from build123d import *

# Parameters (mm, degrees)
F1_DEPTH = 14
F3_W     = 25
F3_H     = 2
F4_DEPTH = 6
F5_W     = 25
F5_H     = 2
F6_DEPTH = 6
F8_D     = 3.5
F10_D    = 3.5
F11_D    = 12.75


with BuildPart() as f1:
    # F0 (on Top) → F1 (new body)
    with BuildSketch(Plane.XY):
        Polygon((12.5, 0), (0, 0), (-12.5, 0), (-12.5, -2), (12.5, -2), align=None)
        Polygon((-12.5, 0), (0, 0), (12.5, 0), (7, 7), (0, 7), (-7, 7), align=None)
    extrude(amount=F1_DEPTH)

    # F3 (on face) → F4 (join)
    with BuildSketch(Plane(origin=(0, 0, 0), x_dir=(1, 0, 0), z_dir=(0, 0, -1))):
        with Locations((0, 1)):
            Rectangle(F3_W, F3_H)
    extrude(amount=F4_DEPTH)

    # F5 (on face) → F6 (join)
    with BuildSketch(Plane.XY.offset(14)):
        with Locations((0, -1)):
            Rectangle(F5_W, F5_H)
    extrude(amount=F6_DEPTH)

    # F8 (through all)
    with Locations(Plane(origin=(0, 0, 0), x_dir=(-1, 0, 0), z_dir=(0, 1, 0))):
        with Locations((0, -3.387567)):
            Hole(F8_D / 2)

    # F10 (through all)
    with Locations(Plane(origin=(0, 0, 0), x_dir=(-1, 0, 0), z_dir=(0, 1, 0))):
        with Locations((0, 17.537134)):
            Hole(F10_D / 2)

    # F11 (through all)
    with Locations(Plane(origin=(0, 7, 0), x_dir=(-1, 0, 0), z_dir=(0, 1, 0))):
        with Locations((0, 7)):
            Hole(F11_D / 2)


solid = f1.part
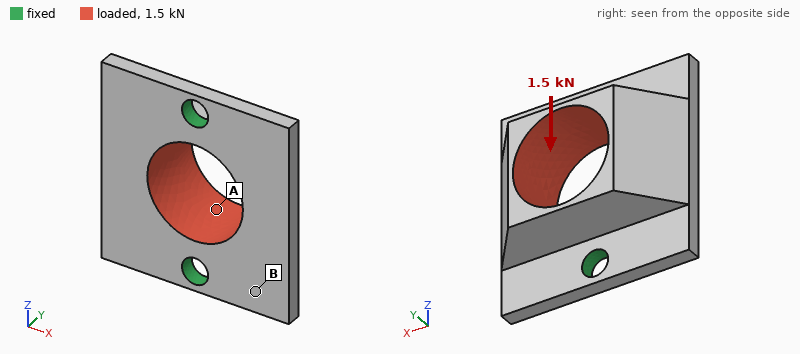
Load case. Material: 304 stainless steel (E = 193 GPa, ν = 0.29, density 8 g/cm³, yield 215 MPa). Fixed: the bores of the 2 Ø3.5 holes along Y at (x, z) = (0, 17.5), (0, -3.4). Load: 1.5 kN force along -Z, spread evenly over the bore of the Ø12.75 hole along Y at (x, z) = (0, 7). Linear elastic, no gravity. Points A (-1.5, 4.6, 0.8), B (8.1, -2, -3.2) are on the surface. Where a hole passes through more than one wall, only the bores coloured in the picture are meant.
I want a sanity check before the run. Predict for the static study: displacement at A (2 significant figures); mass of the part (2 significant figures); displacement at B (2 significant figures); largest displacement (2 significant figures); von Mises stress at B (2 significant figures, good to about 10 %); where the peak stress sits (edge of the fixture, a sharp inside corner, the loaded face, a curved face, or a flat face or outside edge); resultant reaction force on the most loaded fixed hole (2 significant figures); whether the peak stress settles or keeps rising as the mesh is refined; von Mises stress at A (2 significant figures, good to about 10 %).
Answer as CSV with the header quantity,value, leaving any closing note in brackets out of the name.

quantity,value
displacement at A,5.5 µm
mass of the part,16 g
displacement at B,2.7 µm
largest displacement,7.4 µm
von Mises stress at B,14 MPa
where the peak stress sits,edge of the fixture
resultant reaction force on the most loaded fixed hole,810 N
whether the peak stress settles or keeps rising as the mesh is refined,keeps rising
von Mises stress at A,48 MPa
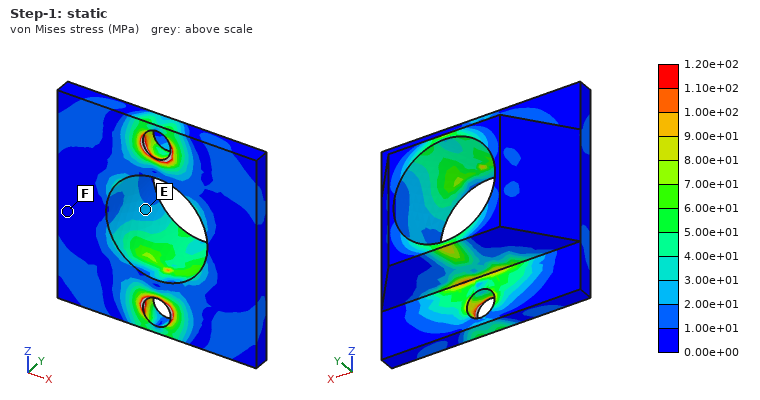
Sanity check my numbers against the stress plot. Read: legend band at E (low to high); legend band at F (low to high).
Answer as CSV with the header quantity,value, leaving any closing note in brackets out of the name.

quantity,value
legend band at E,2.00e+01 to 3.00e+01 MPa
legend band at F,0.00e+00 to 1.00e+01 MPa
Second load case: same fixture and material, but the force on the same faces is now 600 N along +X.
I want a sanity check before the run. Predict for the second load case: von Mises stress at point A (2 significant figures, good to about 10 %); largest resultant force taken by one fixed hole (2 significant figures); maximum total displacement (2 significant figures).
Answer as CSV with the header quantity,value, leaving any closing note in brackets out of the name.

quantity,value
von Mises stress at point A,28 MPa
largest resultant force taken by one fixed hole,300 N
maximum total displacement,12 µm
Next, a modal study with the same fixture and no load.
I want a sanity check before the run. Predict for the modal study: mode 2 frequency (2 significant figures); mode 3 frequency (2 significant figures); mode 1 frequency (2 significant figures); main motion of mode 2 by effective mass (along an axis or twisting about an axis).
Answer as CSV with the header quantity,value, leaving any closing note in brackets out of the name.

quantity,value
mode 2 frequency,16 kHz
mode 3 frequency,22 kHz
mode 1 frequency,7400 Hz
main motion of mode 2 by effective mass,along Y
